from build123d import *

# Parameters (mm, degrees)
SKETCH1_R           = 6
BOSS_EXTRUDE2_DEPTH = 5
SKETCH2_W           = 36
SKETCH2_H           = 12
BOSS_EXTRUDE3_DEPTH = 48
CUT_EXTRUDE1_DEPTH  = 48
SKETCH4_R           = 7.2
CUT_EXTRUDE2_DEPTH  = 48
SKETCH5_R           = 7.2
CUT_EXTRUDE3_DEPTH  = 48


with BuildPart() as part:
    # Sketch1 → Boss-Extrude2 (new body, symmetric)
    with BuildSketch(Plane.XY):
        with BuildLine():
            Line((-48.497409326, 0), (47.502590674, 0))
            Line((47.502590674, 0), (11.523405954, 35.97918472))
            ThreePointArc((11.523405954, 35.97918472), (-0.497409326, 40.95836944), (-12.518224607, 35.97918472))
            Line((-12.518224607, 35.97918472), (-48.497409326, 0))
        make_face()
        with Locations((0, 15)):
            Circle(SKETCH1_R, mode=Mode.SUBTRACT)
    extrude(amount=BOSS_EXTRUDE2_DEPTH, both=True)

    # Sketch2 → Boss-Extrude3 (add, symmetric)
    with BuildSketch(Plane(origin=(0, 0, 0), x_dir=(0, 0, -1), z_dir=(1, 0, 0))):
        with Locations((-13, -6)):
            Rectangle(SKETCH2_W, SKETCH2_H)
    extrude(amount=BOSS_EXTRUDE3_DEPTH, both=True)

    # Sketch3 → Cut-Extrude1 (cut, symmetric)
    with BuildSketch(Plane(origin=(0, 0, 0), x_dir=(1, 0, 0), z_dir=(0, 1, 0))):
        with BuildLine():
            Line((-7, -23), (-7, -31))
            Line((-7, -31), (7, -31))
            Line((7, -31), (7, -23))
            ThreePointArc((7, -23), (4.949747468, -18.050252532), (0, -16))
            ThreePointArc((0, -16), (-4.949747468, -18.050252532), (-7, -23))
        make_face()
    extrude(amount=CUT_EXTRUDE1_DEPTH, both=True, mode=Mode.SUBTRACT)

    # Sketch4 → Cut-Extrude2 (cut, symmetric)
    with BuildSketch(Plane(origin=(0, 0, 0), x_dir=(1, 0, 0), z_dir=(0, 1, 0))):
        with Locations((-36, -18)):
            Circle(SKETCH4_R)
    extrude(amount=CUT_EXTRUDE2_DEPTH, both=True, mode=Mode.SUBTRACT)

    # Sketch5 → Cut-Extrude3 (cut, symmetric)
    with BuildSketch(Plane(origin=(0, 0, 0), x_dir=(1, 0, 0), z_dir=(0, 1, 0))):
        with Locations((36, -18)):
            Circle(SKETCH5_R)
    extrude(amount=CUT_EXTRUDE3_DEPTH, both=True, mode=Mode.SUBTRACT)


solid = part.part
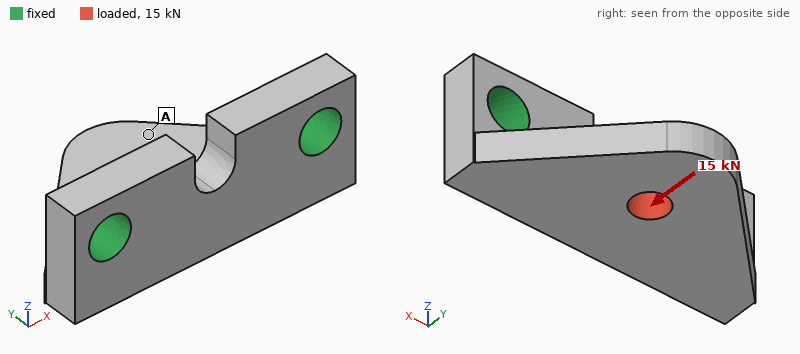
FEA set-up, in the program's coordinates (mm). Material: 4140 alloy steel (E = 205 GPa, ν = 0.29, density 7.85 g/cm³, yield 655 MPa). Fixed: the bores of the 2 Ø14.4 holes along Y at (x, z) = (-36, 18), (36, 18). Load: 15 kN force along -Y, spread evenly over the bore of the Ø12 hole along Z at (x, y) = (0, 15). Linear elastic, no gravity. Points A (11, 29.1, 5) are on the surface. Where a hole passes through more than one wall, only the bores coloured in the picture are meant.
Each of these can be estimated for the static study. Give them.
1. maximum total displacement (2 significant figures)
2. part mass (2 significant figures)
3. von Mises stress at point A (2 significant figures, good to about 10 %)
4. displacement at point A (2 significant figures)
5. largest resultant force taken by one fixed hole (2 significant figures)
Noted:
51 µm
440 g
37 MPa
36 µm
7.8 kN
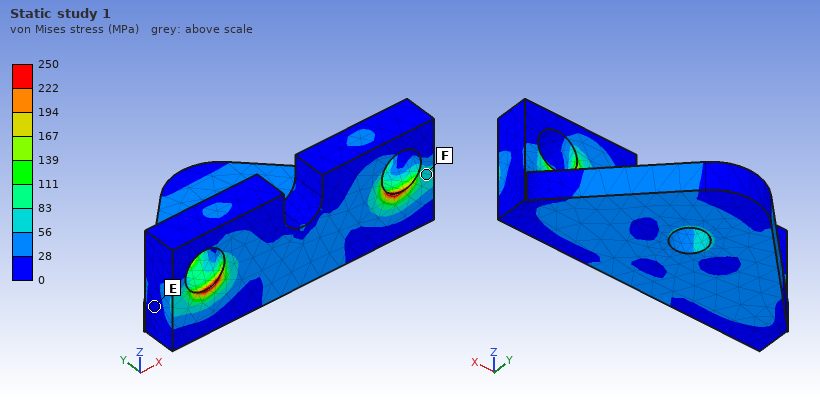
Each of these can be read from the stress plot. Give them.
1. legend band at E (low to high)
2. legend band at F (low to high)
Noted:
0 to 28 MPa
56 to 83 MPa
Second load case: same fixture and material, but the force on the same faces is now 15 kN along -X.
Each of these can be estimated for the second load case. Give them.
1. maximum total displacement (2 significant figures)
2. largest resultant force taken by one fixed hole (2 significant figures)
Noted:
15 µm
9.0 kN
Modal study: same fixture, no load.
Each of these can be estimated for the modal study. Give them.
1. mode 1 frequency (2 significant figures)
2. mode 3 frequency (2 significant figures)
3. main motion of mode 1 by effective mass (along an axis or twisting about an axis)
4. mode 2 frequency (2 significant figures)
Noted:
4200 Hz
11 kHz
along Z
11 kHz
